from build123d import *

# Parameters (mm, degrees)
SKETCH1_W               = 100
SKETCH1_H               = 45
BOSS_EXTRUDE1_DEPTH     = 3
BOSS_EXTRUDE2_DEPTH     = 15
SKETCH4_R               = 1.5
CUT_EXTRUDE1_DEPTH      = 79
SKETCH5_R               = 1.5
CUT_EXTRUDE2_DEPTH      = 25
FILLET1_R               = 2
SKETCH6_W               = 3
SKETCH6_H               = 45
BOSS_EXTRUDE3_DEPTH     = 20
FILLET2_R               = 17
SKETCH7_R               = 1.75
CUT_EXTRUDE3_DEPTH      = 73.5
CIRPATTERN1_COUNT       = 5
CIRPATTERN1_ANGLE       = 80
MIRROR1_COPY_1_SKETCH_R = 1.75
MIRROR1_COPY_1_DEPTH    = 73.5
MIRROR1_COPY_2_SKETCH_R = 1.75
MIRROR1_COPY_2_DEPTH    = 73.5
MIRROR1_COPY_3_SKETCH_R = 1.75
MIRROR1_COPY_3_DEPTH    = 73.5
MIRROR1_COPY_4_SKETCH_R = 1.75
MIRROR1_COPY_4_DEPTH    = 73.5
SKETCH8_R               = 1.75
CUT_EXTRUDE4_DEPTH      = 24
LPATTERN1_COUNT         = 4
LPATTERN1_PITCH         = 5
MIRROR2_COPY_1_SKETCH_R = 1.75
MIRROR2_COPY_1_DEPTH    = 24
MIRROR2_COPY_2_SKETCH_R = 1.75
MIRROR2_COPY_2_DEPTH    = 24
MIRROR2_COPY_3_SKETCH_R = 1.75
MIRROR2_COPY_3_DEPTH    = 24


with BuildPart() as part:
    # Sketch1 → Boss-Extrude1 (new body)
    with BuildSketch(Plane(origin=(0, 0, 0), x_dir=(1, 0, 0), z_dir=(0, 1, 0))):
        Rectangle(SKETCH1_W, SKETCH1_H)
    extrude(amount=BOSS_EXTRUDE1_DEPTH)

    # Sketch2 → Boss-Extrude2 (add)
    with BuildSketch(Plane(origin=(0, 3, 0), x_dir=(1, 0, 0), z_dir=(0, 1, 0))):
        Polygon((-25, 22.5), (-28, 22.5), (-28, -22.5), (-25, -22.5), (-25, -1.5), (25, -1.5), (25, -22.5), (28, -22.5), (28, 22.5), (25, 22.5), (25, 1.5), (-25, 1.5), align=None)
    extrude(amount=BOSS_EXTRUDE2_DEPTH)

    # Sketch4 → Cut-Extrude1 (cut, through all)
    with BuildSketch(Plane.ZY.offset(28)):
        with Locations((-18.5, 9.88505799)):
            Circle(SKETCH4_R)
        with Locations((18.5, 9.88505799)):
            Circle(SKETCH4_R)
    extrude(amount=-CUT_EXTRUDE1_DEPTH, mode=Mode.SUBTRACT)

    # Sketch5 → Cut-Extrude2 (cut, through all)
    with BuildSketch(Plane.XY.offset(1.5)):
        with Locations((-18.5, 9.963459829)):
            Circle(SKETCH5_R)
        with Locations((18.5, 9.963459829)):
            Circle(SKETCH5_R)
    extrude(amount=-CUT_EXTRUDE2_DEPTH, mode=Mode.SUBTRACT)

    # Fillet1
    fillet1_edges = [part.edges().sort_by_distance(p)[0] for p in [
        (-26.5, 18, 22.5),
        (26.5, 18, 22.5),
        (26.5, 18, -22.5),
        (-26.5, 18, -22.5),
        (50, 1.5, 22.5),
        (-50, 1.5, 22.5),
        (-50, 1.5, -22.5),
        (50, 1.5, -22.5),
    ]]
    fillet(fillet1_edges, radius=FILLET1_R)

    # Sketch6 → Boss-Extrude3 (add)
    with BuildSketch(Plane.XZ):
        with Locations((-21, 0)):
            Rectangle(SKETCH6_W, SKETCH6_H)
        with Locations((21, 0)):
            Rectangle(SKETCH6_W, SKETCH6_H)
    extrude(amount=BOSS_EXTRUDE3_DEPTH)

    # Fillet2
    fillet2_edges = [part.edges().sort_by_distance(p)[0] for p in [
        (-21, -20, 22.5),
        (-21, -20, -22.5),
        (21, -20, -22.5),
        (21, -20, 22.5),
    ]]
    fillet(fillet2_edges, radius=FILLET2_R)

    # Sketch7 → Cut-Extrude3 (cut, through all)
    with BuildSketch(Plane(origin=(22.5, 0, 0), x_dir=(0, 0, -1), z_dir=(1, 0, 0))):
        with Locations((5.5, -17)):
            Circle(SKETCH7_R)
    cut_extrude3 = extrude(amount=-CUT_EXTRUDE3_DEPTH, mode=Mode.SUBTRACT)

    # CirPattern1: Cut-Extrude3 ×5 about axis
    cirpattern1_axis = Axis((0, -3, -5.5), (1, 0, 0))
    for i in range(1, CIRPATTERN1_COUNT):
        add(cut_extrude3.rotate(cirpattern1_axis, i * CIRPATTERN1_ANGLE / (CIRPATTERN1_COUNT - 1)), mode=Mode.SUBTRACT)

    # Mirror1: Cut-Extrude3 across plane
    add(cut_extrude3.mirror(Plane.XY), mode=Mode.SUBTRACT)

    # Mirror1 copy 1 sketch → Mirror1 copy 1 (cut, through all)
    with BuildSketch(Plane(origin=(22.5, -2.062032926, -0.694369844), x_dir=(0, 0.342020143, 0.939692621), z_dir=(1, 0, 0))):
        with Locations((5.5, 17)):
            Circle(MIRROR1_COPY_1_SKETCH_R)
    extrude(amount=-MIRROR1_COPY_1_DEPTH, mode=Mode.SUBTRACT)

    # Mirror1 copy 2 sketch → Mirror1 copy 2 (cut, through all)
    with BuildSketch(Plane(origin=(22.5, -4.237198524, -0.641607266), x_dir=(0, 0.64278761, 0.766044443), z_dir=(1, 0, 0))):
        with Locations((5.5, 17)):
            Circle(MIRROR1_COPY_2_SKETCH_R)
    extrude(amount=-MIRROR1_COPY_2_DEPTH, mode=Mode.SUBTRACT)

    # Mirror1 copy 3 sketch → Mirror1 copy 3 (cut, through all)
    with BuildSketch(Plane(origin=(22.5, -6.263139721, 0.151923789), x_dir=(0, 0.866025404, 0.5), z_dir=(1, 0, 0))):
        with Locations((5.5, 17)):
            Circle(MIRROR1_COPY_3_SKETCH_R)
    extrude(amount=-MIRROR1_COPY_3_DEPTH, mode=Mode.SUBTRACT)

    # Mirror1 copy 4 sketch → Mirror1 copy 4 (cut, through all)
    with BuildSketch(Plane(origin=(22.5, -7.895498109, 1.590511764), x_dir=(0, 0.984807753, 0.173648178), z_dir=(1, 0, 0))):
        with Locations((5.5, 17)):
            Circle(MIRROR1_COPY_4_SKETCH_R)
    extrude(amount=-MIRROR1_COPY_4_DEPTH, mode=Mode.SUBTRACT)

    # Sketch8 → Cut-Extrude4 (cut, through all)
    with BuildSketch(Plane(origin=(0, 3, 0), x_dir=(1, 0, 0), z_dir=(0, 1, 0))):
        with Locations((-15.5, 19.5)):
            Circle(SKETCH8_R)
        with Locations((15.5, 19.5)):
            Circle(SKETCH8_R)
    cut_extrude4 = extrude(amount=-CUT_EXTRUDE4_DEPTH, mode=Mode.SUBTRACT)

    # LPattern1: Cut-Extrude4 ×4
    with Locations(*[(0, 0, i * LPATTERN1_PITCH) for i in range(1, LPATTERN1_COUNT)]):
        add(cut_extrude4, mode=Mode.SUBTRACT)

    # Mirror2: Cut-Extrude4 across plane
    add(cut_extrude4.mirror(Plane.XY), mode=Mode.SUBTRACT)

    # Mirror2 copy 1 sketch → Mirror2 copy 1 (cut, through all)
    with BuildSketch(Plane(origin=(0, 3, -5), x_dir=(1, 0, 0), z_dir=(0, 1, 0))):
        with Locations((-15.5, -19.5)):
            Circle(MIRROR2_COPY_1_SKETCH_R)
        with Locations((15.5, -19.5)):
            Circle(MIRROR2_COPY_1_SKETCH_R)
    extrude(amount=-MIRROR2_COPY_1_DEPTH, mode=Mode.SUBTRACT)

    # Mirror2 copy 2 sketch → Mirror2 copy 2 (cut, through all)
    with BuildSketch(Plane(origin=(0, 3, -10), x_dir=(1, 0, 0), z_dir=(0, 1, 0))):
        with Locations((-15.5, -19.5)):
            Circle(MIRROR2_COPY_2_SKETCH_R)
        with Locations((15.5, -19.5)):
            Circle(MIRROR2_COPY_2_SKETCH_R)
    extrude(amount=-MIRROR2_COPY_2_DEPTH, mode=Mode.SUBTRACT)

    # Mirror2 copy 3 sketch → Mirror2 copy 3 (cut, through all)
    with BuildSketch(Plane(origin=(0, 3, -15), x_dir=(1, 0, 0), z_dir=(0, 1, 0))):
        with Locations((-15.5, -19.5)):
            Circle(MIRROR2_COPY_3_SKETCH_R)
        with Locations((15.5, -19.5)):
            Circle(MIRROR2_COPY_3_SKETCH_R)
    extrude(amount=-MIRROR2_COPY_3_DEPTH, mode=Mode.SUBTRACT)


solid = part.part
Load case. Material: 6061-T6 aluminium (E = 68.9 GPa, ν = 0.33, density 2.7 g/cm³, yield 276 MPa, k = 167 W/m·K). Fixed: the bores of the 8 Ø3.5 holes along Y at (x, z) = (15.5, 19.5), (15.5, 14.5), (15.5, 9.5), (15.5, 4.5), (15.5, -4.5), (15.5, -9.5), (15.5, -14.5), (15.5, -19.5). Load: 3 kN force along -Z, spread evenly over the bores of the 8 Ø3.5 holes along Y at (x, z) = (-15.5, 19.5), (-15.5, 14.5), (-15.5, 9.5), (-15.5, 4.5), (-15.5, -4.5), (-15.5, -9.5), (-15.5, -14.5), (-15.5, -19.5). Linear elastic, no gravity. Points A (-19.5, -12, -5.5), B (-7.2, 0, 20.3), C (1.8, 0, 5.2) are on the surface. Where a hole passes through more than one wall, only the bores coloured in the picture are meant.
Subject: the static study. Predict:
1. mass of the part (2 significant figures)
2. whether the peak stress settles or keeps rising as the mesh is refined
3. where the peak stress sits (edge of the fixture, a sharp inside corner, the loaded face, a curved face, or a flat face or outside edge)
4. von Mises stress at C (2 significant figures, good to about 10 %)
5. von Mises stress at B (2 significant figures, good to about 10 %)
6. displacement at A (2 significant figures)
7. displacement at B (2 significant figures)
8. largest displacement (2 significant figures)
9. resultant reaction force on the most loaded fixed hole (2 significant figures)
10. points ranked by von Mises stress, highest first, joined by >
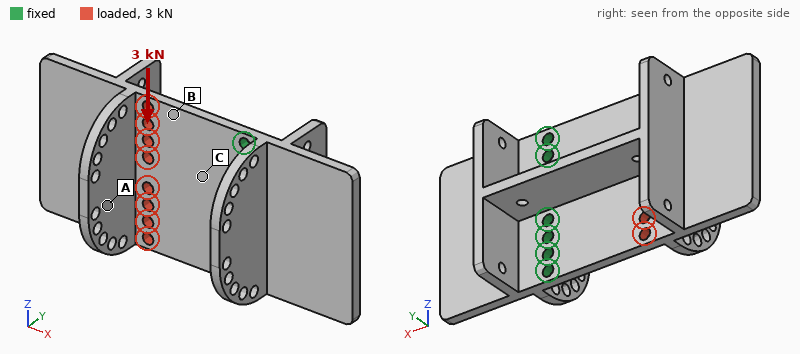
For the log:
63 g
keeps rising
edge of the fixture
55 MPa
25 MPa
60 µm
36 µm
84 µm
1.6 kN
C > B > A
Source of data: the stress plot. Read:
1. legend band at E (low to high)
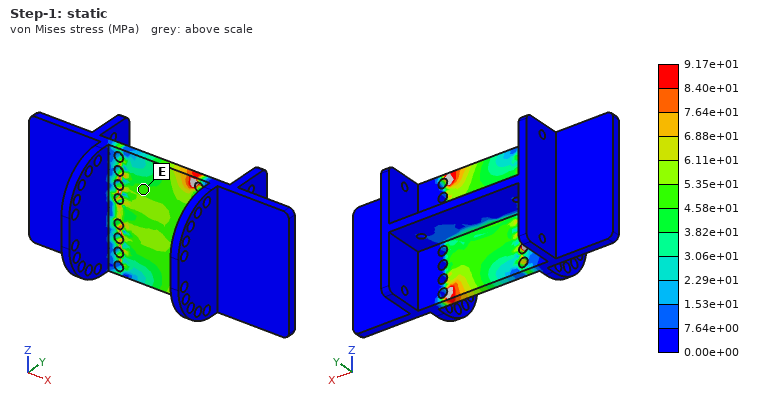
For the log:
4.58e+01 to 5.35e+01 MPa
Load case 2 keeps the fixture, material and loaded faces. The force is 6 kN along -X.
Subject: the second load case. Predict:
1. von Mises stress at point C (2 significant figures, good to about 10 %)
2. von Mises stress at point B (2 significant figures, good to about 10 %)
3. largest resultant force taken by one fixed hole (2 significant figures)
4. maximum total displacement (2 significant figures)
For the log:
45 MPa
44 MPa
910 N
70 µm
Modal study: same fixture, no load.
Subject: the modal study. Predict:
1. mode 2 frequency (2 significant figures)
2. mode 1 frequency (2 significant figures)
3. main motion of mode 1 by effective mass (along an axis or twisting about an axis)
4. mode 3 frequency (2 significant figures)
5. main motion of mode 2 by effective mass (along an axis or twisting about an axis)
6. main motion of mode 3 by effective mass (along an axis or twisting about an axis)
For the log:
1700 Hz
1200 Hz
along Y
3500 Hz
twisting about X
along Y
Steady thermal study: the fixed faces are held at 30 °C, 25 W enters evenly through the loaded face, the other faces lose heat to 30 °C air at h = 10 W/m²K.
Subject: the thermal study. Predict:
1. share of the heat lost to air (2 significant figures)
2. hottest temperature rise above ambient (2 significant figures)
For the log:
8.8 %
27 K
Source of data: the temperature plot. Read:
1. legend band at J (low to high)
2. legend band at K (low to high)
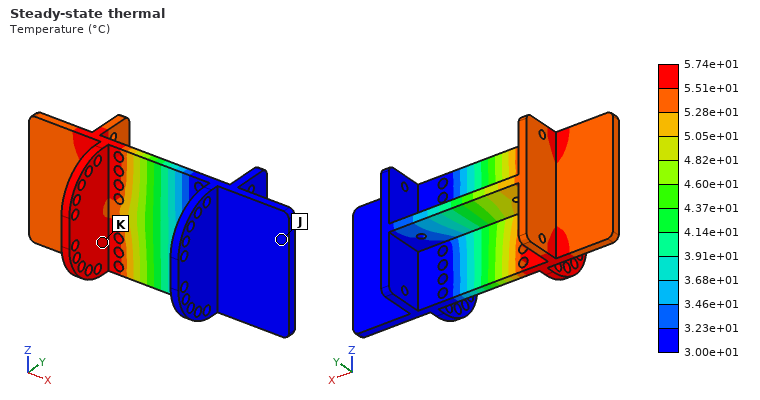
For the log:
3.00e+01 to 3.23e+01 °C
5.51e+01 to 5.74e+01 °C
